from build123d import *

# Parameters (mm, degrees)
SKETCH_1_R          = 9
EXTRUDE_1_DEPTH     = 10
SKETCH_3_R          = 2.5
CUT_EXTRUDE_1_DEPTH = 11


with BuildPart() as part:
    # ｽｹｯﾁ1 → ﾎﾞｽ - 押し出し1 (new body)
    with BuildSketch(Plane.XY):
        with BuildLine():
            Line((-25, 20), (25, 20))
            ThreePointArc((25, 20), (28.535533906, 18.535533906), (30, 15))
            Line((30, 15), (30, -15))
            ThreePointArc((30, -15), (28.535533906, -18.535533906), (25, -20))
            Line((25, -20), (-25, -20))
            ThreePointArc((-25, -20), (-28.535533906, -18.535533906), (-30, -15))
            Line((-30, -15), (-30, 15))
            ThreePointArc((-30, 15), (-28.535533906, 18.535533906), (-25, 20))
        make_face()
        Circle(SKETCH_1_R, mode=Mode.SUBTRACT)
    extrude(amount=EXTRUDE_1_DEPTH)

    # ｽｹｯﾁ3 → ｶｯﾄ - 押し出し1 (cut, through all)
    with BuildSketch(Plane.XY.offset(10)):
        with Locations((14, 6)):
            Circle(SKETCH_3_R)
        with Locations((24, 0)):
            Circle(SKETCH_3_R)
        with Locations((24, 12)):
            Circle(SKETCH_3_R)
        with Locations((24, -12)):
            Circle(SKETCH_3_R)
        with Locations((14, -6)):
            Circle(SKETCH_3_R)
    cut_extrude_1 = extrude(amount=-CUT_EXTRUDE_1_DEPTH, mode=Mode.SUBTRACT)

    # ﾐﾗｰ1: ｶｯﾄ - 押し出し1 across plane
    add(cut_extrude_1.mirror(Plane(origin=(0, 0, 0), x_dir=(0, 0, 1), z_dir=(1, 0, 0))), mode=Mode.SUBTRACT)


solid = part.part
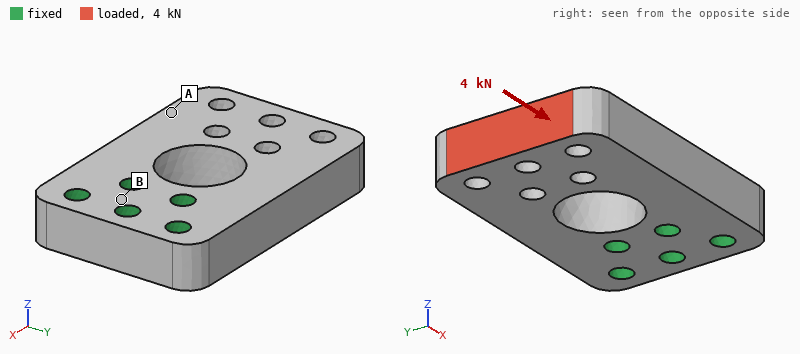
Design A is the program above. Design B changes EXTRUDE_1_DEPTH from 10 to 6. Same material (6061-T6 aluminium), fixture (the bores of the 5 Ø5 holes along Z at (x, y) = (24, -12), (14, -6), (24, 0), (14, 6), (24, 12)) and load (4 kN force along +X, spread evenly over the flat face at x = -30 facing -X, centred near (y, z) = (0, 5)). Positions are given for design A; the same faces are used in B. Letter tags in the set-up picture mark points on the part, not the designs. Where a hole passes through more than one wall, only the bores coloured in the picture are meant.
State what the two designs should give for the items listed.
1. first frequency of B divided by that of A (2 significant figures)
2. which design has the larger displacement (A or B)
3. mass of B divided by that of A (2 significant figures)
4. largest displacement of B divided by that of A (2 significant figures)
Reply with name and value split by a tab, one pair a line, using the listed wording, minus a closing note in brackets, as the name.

first frequency of B divided by that of A	0.64
which design has the larger displacement	B
mass of B divided by that of A	0.60
largest displacement of B divided by that of A	1.7
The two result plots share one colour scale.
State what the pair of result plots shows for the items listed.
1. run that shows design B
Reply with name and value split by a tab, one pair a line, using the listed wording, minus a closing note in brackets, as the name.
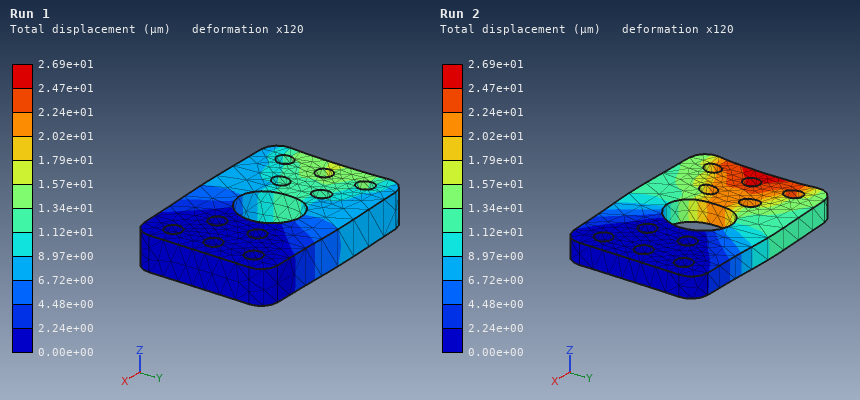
run that shows design B	Run 2
